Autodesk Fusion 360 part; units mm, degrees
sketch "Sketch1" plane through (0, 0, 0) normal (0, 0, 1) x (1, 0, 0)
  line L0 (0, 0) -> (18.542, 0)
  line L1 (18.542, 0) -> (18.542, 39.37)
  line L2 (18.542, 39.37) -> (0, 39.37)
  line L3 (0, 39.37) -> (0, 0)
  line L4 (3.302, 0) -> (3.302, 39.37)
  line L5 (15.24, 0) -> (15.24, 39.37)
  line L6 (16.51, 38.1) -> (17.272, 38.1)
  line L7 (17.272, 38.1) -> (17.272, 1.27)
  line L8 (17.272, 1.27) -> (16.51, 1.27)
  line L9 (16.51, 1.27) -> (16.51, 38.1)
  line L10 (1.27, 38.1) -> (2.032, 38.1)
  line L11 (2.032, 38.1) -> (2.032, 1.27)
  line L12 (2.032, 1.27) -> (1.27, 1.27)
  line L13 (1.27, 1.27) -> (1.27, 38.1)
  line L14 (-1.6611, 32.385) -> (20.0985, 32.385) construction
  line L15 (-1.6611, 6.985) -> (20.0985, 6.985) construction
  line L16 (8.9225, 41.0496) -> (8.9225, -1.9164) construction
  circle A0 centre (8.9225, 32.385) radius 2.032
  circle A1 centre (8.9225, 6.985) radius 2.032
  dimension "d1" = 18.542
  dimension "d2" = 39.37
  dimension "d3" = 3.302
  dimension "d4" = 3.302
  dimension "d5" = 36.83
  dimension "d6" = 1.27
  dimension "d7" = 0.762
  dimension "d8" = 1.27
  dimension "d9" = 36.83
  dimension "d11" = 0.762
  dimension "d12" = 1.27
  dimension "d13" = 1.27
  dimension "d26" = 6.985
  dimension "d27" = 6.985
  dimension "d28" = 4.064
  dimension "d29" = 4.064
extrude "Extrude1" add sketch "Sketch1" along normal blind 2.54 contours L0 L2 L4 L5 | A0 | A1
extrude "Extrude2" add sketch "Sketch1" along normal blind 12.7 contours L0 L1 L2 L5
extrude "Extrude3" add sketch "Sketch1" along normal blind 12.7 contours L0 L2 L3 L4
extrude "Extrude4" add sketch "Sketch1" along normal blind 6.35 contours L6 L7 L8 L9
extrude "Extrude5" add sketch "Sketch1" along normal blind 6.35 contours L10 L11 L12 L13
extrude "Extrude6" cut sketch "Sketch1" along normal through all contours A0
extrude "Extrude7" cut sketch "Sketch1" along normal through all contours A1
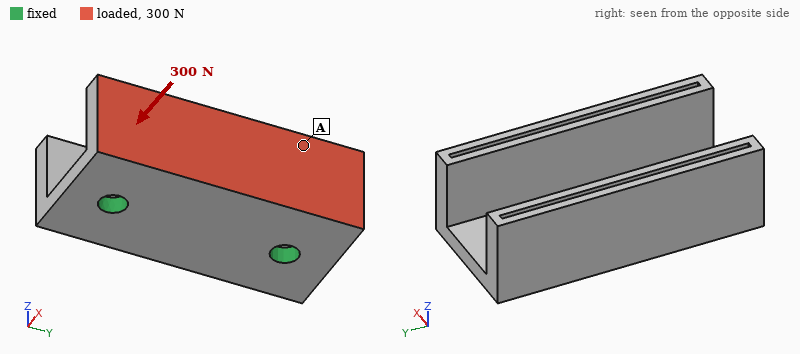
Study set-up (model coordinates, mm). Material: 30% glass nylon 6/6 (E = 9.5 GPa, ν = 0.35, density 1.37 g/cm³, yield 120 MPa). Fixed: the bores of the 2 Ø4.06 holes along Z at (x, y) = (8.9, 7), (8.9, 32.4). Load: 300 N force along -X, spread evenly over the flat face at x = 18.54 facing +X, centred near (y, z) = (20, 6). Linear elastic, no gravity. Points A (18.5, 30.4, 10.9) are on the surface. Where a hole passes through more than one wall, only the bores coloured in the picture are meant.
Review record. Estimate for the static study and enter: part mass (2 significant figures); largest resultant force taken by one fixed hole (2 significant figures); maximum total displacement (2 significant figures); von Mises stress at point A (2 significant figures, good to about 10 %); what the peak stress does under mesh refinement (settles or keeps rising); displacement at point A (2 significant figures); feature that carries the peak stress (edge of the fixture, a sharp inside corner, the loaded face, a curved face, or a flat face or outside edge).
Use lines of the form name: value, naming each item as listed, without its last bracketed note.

part mass: 5.6 g
largest resultant force taken by one fixed hole: 150 N
maximum total displacement: 0.36 mm
von Mises stress at point A: 8.4 MPa
what the peak stress does under mesh refinement: keeps rising
displacement at point A: 0.29 mm
feature that carries the peak stress: edge of the fixture
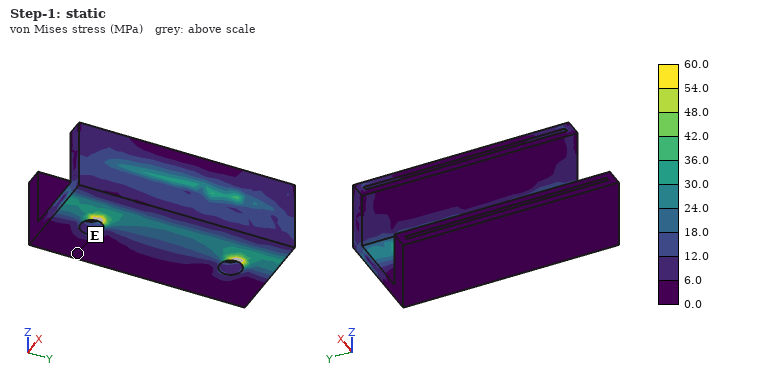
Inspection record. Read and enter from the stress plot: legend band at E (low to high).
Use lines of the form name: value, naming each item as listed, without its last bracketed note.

legend band at E: 0.0 to 6.0 MPa
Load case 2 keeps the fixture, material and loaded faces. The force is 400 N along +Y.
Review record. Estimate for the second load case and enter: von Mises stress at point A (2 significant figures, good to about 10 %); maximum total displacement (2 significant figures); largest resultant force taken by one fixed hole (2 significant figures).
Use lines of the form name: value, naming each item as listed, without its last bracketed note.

von Mises stress at point A: 3.4 MPa
maximum total displacement: 75 µm
largest resultant force taken by one fixed hole: 250 N
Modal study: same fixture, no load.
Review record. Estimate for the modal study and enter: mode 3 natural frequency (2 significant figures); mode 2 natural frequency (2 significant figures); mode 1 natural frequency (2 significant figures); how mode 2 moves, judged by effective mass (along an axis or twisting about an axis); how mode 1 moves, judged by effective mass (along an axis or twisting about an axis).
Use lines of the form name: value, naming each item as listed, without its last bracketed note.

mode 3 natural frequency: 5400 Hz
mode 2 natural frequency: 4400 Hz
mode 1 natural frequency: 3900 Hz
how mode 2 moves, judged by effective mass: along Z
how mode 1 moves, judged by effective mass: along X
